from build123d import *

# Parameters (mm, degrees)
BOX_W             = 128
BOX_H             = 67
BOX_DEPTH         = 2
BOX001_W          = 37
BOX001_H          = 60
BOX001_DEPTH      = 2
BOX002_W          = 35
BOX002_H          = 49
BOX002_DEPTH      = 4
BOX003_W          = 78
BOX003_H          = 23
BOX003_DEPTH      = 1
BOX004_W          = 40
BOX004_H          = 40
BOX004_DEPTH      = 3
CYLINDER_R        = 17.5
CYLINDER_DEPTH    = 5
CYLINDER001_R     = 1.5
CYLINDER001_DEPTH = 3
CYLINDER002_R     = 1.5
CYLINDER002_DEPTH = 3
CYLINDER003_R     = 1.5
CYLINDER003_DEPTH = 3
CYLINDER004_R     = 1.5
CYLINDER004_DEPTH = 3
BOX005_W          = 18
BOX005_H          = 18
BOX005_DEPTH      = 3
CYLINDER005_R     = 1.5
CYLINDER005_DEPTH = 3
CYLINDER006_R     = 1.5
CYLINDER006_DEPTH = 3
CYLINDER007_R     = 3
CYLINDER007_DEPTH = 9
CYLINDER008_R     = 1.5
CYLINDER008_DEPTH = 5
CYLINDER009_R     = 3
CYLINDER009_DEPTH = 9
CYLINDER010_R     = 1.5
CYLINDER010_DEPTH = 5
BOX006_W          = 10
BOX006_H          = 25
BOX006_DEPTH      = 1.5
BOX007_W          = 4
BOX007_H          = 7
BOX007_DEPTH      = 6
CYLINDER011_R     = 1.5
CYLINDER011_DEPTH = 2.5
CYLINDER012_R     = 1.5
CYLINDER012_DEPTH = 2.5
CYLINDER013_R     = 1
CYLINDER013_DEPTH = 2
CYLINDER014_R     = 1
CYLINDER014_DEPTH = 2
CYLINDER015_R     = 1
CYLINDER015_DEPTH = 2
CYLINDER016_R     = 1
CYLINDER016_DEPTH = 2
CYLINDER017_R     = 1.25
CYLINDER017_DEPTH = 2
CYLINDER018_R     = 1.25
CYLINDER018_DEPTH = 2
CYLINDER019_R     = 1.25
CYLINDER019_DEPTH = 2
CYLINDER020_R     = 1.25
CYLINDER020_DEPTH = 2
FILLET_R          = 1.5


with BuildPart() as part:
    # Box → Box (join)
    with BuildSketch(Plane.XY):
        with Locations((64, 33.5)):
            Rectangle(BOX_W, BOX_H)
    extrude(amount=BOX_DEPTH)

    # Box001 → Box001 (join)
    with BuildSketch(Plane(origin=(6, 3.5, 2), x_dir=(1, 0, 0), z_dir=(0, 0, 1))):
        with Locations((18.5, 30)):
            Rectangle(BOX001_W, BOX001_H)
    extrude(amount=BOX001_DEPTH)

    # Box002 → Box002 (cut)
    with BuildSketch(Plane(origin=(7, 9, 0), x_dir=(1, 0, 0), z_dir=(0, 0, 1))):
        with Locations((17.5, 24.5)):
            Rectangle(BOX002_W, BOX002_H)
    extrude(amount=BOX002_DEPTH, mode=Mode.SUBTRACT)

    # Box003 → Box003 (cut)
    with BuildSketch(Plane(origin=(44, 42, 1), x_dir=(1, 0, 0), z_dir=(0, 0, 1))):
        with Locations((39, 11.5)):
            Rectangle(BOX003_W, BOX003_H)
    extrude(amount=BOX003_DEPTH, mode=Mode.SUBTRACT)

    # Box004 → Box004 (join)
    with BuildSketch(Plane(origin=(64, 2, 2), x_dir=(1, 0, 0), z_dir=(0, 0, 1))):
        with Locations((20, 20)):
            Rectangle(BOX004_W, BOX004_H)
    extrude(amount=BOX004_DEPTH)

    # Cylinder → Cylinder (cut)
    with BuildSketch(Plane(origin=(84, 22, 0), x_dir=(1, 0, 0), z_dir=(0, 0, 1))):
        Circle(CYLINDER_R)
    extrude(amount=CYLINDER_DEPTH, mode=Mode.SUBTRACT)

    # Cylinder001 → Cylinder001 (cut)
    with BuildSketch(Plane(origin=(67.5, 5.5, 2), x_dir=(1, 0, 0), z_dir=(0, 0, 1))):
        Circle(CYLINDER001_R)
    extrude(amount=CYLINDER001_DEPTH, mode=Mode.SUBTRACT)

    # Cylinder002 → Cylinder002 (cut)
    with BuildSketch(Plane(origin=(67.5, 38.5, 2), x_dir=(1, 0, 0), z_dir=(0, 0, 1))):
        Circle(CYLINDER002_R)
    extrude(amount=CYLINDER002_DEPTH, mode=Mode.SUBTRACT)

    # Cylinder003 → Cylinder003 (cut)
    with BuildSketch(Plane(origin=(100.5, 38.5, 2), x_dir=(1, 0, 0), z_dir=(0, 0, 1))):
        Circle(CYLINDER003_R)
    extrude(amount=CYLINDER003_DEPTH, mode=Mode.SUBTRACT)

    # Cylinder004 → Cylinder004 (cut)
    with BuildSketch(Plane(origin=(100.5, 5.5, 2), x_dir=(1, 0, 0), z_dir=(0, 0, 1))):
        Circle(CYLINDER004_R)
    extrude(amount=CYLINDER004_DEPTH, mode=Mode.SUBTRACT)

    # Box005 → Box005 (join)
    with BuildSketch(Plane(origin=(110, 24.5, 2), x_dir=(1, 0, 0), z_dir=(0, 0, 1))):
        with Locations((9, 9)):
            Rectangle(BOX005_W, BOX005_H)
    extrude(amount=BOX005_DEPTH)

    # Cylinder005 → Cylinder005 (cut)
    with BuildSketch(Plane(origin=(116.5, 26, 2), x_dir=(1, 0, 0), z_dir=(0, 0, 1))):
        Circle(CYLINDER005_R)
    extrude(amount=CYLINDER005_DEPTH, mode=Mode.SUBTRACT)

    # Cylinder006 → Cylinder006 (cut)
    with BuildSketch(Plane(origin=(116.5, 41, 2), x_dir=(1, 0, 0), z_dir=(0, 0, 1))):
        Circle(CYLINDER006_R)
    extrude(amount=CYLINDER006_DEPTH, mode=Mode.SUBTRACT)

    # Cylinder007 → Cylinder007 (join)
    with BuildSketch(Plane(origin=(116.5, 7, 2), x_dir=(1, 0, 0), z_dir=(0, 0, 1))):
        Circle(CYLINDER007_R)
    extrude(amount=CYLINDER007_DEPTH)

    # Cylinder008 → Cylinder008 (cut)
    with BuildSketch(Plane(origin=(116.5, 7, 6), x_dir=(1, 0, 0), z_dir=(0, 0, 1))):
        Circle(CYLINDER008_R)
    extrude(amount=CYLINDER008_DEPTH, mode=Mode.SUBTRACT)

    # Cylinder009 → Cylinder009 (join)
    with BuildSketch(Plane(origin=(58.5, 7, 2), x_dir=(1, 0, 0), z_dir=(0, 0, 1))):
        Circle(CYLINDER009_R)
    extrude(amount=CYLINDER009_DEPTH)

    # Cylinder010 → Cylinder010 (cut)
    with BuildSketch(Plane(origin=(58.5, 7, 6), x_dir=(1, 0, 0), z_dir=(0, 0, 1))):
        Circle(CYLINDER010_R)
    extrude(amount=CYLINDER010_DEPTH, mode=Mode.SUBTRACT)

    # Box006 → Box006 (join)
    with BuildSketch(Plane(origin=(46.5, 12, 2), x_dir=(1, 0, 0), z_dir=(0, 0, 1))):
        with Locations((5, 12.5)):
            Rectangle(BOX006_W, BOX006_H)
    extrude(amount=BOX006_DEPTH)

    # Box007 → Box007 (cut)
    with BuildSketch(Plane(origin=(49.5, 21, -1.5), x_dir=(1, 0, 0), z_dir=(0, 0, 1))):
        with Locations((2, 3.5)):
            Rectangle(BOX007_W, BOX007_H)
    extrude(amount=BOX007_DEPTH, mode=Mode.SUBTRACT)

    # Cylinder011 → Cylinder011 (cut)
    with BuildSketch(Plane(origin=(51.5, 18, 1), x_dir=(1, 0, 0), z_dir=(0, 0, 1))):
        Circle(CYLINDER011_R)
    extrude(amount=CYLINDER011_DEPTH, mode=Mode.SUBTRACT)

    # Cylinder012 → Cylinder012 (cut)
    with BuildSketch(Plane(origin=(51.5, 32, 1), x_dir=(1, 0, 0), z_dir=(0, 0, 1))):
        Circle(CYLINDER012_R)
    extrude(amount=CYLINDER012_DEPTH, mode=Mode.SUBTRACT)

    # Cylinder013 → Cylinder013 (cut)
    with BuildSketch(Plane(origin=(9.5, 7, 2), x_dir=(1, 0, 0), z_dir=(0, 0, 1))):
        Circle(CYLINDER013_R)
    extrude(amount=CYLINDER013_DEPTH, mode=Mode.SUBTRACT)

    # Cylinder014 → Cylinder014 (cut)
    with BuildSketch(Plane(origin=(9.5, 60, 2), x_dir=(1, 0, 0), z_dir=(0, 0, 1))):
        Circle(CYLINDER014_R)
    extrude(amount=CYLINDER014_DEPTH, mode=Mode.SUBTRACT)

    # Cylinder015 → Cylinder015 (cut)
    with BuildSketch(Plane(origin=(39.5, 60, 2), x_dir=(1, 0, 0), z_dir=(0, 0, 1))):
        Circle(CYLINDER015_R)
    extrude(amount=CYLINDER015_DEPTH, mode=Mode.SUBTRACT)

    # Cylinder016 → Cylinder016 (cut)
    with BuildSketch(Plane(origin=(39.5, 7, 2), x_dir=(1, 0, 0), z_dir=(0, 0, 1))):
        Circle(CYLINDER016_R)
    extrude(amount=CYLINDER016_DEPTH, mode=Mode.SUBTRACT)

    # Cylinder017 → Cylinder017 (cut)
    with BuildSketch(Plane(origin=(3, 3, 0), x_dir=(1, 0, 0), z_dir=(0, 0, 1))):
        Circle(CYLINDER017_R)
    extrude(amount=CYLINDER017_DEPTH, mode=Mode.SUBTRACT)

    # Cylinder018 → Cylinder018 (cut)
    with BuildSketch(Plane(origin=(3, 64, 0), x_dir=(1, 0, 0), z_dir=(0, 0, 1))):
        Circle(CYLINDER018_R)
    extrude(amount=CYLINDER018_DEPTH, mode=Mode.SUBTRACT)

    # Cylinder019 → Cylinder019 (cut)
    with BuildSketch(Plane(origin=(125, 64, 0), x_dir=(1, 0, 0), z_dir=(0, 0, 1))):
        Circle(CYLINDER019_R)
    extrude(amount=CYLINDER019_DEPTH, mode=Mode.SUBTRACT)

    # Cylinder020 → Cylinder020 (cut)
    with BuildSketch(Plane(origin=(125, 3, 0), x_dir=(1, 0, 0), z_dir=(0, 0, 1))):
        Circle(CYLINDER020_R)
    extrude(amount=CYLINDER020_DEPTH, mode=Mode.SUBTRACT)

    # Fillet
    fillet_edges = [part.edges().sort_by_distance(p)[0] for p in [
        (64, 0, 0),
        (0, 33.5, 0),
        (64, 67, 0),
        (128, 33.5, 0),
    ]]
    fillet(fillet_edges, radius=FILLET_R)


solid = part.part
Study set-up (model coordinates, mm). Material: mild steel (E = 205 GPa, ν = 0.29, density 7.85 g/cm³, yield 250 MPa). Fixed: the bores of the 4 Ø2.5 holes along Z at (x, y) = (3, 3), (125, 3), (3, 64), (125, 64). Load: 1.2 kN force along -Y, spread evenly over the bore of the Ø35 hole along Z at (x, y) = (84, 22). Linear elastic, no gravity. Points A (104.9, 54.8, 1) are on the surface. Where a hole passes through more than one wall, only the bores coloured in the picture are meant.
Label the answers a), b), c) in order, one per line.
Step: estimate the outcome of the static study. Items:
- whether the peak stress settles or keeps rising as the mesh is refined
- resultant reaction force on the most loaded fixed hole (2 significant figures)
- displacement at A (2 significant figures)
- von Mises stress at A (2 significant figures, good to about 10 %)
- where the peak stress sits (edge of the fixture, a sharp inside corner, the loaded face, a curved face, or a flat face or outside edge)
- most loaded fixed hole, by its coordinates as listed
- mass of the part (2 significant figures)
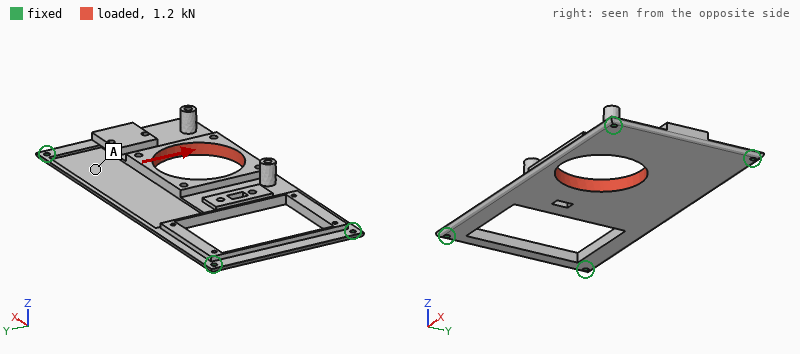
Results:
a) keeps rising
b) 850 N
c) 24 µm
d) 27 MPa
e) edge of the fixture
f) (125, 3)
g) 110 g
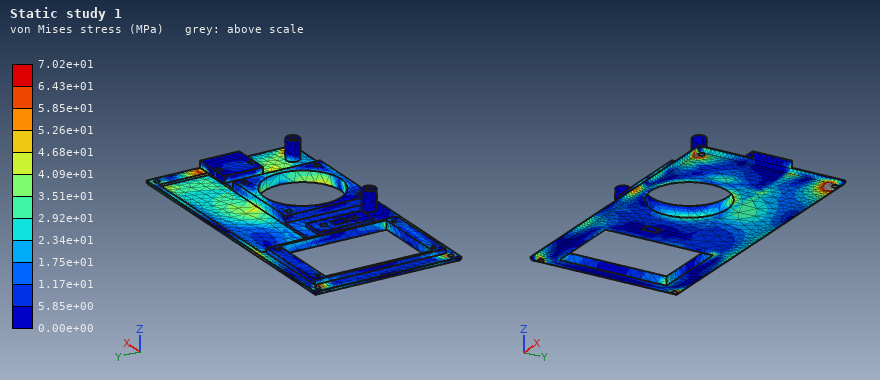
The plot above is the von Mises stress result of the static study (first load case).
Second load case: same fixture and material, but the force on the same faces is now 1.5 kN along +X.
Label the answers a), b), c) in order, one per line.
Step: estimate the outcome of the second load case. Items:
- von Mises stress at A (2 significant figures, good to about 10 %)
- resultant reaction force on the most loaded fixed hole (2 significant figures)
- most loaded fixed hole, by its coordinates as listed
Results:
a) 19 MPa
b) 690 N
c) (125, 3)
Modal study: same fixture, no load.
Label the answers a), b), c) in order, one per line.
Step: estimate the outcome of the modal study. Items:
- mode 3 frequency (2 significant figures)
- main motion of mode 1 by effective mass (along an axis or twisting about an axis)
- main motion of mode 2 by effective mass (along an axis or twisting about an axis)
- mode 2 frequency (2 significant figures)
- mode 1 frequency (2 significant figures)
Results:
a) 1700 Hz
b) along Z
c) twisting about X
d) 1100 Hz
e) 600 Hz
